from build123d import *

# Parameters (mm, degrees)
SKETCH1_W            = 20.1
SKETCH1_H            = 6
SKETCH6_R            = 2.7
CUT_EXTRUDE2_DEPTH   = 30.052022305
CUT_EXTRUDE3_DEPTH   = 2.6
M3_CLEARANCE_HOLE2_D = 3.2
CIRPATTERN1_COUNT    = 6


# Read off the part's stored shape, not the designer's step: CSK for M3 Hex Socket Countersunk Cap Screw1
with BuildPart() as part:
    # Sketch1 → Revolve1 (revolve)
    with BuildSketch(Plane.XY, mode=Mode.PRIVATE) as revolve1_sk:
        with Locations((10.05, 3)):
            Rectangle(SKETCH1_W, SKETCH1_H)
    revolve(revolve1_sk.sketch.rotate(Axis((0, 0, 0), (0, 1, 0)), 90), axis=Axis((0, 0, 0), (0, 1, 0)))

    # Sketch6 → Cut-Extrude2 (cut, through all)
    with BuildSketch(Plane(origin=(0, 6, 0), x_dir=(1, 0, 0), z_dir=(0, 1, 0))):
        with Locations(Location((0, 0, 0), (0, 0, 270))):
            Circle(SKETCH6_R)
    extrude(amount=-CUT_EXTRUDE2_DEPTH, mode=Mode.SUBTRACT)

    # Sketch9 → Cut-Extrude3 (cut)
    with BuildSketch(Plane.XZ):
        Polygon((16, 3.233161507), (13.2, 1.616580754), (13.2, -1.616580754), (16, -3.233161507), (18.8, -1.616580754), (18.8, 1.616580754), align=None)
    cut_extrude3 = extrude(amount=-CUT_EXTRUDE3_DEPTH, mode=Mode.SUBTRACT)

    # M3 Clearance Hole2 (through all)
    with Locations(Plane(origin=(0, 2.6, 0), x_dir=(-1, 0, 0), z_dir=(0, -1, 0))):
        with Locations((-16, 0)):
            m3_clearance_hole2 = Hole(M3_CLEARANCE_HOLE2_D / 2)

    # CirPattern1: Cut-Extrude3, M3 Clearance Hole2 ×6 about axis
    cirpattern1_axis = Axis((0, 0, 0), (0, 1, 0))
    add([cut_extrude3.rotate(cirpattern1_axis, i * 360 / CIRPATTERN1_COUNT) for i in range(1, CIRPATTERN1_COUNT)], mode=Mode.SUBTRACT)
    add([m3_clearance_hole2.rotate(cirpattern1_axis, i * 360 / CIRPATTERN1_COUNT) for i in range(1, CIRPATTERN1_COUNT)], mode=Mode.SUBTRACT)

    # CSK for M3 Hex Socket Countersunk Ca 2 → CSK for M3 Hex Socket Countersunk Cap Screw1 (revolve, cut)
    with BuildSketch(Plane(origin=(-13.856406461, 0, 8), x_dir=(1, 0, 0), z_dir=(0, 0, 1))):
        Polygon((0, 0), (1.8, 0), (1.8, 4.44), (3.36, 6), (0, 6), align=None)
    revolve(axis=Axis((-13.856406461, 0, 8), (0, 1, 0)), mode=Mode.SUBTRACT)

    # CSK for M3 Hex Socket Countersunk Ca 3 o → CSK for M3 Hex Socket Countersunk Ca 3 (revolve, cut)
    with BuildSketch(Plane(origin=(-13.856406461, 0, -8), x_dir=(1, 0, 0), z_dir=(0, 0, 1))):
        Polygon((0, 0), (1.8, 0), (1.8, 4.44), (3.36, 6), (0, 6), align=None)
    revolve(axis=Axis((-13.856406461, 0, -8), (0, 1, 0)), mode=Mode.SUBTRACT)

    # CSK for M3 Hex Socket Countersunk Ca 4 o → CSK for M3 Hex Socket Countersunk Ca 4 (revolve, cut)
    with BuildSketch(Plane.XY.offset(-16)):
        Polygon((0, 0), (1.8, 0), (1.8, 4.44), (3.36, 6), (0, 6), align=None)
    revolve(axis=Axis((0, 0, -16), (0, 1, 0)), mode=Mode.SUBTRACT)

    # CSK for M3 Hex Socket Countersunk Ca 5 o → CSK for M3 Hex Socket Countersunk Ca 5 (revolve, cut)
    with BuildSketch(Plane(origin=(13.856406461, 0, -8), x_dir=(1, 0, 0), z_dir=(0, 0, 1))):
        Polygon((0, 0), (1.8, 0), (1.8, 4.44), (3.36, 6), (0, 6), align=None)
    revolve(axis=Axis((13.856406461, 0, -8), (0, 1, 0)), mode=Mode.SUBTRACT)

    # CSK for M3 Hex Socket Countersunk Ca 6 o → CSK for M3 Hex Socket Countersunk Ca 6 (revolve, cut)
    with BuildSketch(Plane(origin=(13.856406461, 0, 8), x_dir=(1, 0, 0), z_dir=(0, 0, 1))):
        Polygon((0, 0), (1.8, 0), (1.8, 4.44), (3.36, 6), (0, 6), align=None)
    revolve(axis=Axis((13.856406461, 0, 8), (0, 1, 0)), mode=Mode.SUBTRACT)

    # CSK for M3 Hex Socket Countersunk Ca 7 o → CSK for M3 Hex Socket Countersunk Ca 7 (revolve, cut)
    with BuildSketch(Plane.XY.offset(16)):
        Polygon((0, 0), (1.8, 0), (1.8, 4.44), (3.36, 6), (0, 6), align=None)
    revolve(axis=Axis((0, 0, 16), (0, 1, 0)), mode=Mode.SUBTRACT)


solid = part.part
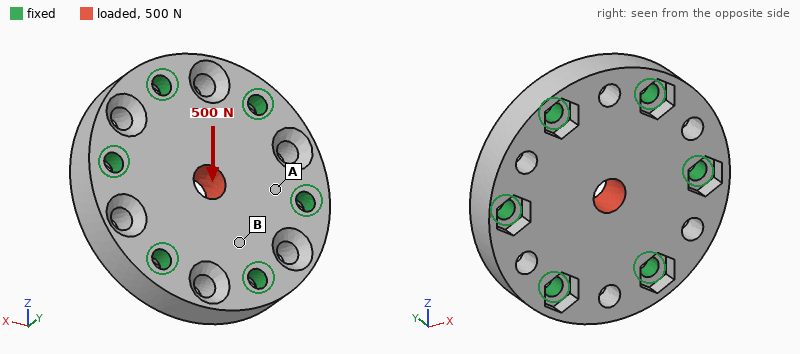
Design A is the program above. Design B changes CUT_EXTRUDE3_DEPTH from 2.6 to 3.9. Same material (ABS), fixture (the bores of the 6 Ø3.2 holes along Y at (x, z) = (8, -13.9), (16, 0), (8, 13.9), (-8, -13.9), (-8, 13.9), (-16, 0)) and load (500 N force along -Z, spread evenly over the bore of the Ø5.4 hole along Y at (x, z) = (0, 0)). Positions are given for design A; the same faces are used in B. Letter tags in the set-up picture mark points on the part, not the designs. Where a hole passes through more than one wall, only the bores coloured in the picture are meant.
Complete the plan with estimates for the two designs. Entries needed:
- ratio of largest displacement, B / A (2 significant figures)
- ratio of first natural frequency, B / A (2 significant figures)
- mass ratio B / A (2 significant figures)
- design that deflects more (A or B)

1.2
0.91
0.98
B
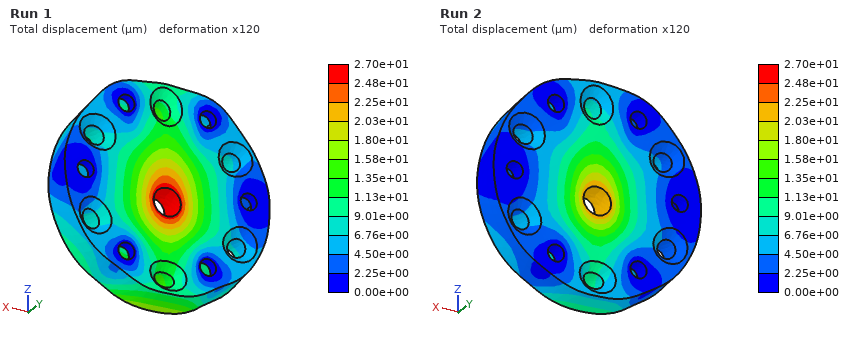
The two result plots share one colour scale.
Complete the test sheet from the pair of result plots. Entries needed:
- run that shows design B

Run 1
